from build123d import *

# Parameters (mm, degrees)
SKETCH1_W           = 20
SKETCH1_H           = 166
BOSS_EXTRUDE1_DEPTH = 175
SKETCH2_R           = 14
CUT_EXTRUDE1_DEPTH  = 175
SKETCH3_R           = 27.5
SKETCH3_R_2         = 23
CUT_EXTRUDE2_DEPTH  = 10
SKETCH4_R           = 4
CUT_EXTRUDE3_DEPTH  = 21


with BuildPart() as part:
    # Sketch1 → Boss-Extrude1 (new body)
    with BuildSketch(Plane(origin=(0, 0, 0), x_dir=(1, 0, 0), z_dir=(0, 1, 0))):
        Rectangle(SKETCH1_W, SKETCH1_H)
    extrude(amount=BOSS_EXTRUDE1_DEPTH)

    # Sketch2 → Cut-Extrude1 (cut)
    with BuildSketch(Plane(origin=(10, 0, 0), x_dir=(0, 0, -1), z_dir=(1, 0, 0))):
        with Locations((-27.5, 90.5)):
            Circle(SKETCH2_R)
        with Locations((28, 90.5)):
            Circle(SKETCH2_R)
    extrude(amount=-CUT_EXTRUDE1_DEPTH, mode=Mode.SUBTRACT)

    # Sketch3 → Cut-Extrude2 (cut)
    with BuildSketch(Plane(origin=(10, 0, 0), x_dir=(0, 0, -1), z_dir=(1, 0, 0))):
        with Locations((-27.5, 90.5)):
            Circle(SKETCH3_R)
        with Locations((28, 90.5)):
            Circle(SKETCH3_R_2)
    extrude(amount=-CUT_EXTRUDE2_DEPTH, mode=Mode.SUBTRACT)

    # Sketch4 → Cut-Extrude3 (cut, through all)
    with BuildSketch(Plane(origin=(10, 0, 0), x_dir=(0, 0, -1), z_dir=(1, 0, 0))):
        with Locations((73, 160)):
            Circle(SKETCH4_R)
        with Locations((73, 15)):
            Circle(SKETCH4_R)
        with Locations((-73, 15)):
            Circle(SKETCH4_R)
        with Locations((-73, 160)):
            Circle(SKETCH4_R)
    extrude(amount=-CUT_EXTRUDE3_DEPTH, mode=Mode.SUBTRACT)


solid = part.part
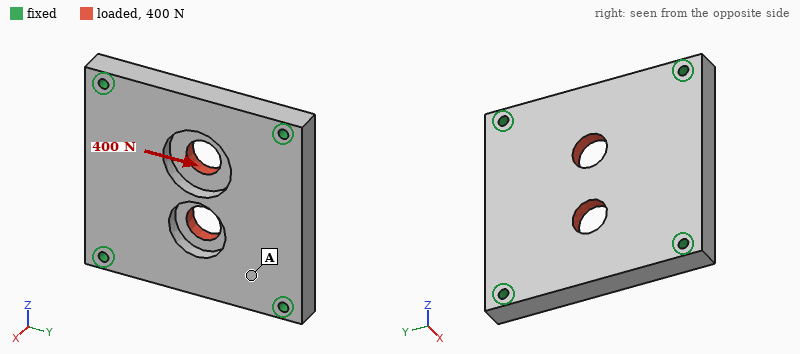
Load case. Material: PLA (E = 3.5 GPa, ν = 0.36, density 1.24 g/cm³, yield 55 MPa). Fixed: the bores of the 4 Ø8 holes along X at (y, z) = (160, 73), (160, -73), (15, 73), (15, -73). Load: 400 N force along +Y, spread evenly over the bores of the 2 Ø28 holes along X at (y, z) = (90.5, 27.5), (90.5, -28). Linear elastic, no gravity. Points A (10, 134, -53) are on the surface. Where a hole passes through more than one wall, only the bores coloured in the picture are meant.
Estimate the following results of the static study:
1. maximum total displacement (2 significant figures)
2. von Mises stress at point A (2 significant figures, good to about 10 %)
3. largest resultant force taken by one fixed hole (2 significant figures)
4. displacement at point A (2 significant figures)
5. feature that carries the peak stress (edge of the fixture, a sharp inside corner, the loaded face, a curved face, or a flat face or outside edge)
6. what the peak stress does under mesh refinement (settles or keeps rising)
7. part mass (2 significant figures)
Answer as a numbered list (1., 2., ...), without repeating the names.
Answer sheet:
1. 5.6 µm
2. 0.11 MPa
3. 110 N
4. 2.0 µm
5. edge of the fixture
6. keeps rising
7. 650 g
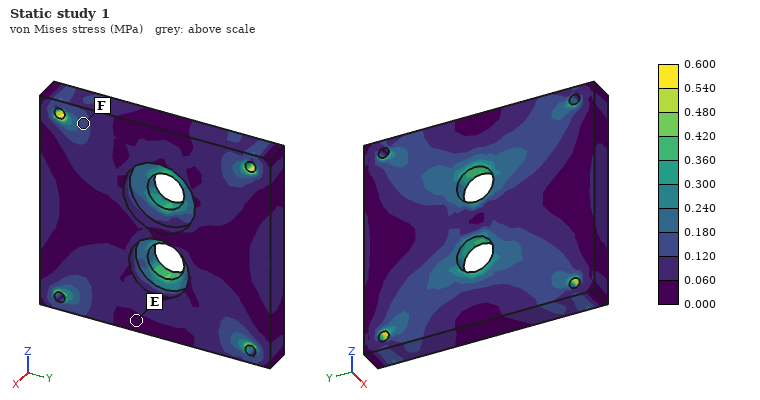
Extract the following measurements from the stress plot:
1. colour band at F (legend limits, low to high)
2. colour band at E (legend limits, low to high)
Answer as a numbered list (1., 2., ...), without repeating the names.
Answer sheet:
1. 0.120 to 0.180 MPa
2. 0.000 to 0.060 MPa
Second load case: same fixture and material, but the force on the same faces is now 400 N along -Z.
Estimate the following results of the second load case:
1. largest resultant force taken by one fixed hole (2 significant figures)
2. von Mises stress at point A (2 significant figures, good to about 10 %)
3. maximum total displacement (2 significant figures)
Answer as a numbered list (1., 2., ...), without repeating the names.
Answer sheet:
1. 120 N
2. 0.11 MPa
3. 7.1 µm
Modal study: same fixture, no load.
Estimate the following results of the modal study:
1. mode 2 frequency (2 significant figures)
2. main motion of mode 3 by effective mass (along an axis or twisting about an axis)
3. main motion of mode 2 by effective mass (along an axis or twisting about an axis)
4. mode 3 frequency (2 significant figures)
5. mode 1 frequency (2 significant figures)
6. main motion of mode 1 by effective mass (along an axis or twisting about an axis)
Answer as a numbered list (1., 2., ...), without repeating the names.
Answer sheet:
1. 1400 Hz
2. twisting about Y
3. twisting about Z
4. 1500 Hz
5. 900 Hz
6. along X
